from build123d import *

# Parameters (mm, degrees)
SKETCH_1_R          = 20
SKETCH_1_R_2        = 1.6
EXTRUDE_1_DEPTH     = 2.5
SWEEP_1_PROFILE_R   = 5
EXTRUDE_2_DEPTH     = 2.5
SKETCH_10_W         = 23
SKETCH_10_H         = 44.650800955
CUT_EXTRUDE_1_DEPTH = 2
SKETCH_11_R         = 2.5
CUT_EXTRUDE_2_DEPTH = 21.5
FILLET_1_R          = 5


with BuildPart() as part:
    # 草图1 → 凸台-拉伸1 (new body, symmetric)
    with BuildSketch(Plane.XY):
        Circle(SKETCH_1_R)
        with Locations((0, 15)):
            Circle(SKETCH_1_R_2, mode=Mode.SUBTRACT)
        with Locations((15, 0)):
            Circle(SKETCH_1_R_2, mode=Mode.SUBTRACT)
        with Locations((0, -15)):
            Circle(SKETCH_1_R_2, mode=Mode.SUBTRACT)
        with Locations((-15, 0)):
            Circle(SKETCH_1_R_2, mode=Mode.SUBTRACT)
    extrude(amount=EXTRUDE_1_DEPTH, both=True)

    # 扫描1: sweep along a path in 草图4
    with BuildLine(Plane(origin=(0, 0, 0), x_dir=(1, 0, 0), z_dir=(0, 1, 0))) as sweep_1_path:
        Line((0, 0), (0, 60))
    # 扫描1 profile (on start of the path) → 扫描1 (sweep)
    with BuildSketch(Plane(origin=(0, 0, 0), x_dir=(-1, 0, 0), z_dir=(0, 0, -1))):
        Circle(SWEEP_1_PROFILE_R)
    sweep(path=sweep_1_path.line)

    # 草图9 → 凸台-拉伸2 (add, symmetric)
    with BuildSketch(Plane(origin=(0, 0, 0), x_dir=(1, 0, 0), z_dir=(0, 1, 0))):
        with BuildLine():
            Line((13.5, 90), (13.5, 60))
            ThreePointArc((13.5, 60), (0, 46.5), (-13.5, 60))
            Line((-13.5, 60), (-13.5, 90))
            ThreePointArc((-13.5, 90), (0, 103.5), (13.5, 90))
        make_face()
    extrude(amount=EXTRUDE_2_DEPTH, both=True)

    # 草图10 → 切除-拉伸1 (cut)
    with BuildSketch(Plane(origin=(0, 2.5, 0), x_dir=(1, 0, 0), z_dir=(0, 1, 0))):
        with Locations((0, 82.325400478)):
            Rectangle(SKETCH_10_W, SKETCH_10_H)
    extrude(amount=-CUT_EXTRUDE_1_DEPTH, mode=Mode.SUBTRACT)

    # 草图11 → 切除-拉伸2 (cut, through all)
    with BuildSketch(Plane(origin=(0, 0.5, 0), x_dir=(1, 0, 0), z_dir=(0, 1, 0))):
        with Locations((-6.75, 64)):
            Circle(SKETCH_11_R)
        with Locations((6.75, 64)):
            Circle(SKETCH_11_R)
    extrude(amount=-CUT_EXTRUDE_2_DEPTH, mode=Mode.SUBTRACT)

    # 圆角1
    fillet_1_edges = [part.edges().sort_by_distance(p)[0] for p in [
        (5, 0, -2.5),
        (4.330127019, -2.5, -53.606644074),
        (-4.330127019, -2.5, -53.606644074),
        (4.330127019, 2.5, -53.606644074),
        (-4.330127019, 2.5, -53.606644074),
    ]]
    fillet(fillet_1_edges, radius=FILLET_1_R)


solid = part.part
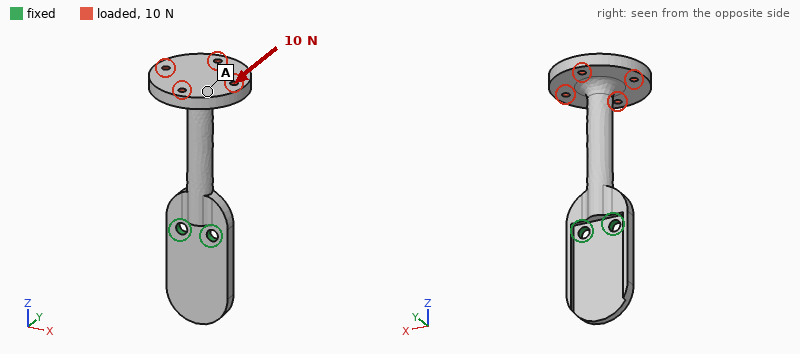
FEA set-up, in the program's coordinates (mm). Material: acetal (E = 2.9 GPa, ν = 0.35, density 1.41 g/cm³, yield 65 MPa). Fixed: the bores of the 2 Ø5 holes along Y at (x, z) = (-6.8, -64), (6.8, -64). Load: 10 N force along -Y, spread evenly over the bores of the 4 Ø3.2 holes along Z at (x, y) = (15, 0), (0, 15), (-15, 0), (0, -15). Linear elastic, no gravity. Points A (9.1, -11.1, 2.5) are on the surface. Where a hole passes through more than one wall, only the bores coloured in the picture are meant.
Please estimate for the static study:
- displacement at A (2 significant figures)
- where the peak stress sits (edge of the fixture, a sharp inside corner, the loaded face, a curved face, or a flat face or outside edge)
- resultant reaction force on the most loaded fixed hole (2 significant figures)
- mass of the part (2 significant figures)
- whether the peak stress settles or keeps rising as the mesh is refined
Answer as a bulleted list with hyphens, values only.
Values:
- 1.2 mm
- edge of the fixture
- 6.0 N
- 21 g
- keeps rising
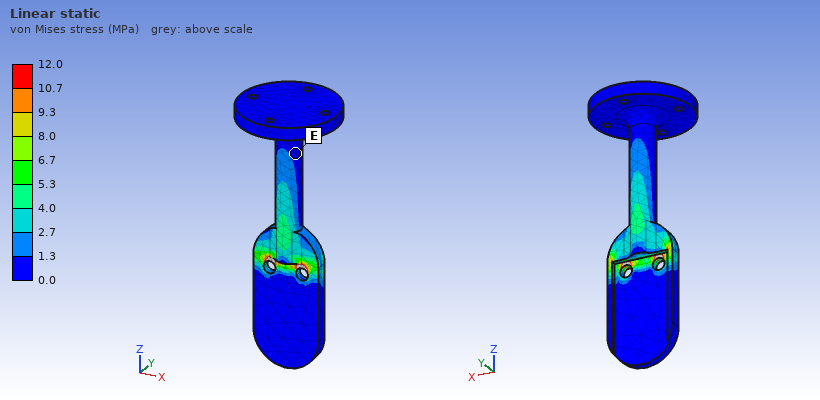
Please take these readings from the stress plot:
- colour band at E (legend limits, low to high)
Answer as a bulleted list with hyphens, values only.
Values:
- 0.0 to 1.3 MPa
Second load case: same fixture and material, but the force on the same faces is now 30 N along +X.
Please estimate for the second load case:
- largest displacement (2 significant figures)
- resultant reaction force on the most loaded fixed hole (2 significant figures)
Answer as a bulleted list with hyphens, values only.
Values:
- 1.2 mm
- 120 N
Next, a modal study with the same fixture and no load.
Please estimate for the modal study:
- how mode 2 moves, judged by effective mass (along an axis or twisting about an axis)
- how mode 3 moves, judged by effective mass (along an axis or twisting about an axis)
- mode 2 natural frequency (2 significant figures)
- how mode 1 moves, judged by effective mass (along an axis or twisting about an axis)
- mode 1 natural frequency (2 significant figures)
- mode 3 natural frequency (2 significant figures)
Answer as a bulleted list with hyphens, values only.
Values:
- along X
- twisting about Z
- 270 Hz
- along Y
- 150 Hz
- 530 Hz
